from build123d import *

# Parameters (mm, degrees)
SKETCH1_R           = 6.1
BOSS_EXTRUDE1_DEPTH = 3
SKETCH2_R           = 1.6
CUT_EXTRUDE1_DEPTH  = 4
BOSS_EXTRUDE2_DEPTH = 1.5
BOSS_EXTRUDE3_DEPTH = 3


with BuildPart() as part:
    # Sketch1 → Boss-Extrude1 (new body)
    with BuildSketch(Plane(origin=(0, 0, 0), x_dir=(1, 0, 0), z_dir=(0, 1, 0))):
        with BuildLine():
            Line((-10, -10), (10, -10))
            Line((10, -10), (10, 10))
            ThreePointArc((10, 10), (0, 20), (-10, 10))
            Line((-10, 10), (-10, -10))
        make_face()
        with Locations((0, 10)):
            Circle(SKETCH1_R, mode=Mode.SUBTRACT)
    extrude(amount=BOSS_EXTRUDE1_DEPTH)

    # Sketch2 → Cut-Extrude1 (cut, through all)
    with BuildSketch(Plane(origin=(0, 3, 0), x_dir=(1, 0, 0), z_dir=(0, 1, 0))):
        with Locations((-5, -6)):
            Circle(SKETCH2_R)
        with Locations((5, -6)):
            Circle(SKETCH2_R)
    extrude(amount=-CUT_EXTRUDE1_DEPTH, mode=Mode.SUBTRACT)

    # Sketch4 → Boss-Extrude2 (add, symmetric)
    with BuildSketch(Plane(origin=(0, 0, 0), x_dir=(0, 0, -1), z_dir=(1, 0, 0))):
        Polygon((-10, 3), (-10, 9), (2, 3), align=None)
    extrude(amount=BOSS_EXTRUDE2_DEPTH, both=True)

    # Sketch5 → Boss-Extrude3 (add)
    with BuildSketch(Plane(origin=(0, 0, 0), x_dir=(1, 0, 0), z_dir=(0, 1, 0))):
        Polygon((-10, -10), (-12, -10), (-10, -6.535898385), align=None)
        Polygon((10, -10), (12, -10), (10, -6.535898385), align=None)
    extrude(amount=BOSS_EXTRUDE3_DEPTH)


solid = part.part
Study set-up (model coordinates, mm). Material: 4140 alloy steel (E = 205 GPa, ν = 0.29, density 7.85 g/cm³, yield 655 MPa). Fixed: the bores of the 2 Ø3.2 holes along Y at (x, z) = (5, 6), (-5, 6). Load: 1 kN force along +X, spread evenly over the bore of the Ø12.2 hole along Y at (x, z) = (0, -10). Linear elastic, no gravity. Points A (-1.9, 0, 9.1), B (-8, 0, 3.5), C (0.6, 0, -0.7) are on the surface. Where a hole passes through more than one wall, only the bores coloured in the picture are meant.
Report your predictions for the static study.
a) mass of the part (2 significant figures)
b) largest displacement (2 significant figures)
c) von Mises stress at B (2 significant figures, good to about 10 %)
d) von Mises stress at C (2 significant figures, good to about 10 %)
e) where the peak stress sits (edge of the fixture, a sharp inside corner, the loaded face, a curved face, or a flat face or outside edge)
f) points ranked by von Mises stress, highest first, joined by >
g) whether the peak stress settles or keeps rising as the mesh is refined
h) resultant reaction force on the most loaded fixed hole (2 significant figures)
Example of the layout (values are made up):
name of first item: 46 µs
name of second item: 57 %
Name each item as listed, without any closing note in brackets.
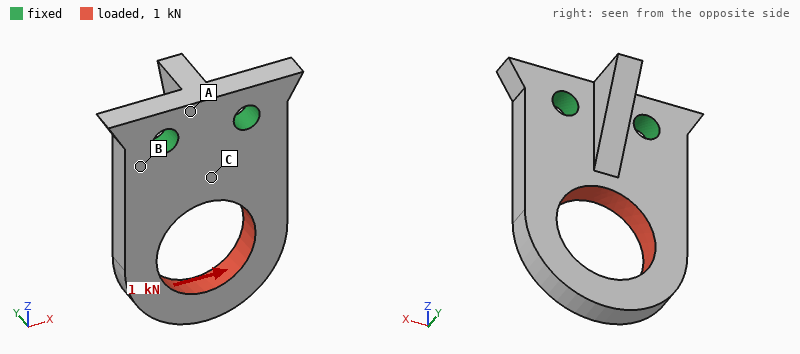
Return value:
mass of the part: 11 g
largest displacement: 26 µm
von Mises stress at B: 47 MPa
von Mises stress at C: 85 MPa
where the peak stress sits: edge of the fixture
points ranked by von Mises stress, highest first, joined by >: C > B > A
whether the peak stress settles or keeps rising as the mesh is refined: keeps rising
resultant reaction force on the most loaded fixed hole: 1.3 kN
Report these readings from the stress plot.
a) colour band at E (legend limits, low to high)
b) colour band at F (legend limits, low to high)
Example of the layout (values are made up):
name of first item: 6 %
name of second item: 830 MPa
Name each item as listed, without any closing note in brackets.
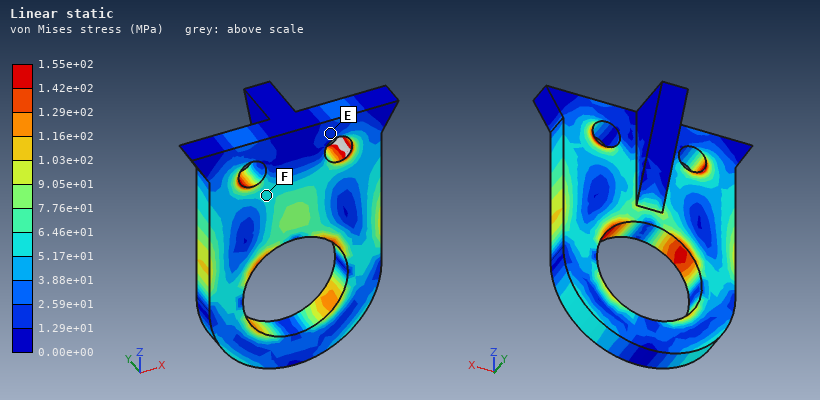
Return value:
colour band at E: 1.29e+01 to 2.59e+01 MPa
colour band at F: 5.17e+01 to 6.46e+01 MPa
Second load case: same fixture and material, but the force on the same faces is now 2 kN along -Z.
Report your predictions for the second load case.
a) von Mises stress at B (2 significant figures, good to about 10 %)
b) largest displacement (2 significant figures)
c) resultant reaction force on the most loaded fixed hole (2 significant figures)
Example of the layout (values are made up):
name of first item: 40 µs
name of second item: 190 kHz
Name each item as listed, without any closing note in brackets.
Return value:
von Mises stress at B: 40 MPa
largest displacement: 9.6 µm
resultant reaction force on the most loaded fixed hole: 1.0 kN
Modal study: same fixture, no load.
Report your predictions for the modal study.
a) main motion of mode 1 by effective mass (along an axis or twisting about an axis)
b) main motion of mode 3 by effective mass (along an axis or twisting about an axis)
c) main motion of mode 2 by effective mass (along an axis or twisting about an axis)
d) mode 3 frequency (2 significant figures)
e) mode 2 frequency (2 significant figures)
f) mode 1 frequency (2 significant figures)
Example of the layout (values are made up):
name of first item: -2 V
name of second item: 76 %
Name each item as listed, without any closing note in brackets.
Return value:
main motion of mode 1 by effective mass: along Y
main motion of mode 3 by effective mass: along X
main motion of mode 2 by effective mass: twisting about Z
mode 3 frequency: 16 kHz
mode 2 frequency: 12 kHz
mode 1 frequency: 5000 Hz
